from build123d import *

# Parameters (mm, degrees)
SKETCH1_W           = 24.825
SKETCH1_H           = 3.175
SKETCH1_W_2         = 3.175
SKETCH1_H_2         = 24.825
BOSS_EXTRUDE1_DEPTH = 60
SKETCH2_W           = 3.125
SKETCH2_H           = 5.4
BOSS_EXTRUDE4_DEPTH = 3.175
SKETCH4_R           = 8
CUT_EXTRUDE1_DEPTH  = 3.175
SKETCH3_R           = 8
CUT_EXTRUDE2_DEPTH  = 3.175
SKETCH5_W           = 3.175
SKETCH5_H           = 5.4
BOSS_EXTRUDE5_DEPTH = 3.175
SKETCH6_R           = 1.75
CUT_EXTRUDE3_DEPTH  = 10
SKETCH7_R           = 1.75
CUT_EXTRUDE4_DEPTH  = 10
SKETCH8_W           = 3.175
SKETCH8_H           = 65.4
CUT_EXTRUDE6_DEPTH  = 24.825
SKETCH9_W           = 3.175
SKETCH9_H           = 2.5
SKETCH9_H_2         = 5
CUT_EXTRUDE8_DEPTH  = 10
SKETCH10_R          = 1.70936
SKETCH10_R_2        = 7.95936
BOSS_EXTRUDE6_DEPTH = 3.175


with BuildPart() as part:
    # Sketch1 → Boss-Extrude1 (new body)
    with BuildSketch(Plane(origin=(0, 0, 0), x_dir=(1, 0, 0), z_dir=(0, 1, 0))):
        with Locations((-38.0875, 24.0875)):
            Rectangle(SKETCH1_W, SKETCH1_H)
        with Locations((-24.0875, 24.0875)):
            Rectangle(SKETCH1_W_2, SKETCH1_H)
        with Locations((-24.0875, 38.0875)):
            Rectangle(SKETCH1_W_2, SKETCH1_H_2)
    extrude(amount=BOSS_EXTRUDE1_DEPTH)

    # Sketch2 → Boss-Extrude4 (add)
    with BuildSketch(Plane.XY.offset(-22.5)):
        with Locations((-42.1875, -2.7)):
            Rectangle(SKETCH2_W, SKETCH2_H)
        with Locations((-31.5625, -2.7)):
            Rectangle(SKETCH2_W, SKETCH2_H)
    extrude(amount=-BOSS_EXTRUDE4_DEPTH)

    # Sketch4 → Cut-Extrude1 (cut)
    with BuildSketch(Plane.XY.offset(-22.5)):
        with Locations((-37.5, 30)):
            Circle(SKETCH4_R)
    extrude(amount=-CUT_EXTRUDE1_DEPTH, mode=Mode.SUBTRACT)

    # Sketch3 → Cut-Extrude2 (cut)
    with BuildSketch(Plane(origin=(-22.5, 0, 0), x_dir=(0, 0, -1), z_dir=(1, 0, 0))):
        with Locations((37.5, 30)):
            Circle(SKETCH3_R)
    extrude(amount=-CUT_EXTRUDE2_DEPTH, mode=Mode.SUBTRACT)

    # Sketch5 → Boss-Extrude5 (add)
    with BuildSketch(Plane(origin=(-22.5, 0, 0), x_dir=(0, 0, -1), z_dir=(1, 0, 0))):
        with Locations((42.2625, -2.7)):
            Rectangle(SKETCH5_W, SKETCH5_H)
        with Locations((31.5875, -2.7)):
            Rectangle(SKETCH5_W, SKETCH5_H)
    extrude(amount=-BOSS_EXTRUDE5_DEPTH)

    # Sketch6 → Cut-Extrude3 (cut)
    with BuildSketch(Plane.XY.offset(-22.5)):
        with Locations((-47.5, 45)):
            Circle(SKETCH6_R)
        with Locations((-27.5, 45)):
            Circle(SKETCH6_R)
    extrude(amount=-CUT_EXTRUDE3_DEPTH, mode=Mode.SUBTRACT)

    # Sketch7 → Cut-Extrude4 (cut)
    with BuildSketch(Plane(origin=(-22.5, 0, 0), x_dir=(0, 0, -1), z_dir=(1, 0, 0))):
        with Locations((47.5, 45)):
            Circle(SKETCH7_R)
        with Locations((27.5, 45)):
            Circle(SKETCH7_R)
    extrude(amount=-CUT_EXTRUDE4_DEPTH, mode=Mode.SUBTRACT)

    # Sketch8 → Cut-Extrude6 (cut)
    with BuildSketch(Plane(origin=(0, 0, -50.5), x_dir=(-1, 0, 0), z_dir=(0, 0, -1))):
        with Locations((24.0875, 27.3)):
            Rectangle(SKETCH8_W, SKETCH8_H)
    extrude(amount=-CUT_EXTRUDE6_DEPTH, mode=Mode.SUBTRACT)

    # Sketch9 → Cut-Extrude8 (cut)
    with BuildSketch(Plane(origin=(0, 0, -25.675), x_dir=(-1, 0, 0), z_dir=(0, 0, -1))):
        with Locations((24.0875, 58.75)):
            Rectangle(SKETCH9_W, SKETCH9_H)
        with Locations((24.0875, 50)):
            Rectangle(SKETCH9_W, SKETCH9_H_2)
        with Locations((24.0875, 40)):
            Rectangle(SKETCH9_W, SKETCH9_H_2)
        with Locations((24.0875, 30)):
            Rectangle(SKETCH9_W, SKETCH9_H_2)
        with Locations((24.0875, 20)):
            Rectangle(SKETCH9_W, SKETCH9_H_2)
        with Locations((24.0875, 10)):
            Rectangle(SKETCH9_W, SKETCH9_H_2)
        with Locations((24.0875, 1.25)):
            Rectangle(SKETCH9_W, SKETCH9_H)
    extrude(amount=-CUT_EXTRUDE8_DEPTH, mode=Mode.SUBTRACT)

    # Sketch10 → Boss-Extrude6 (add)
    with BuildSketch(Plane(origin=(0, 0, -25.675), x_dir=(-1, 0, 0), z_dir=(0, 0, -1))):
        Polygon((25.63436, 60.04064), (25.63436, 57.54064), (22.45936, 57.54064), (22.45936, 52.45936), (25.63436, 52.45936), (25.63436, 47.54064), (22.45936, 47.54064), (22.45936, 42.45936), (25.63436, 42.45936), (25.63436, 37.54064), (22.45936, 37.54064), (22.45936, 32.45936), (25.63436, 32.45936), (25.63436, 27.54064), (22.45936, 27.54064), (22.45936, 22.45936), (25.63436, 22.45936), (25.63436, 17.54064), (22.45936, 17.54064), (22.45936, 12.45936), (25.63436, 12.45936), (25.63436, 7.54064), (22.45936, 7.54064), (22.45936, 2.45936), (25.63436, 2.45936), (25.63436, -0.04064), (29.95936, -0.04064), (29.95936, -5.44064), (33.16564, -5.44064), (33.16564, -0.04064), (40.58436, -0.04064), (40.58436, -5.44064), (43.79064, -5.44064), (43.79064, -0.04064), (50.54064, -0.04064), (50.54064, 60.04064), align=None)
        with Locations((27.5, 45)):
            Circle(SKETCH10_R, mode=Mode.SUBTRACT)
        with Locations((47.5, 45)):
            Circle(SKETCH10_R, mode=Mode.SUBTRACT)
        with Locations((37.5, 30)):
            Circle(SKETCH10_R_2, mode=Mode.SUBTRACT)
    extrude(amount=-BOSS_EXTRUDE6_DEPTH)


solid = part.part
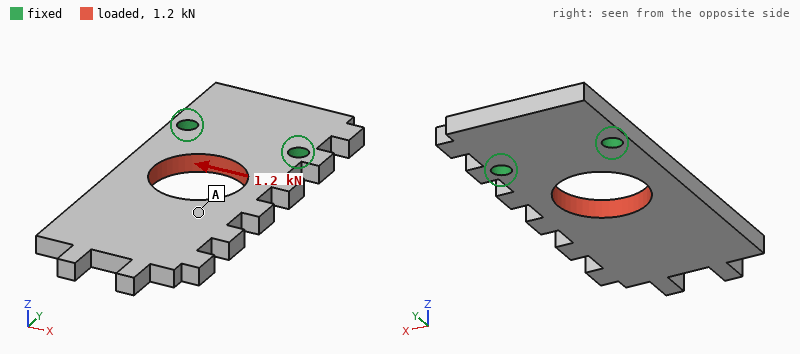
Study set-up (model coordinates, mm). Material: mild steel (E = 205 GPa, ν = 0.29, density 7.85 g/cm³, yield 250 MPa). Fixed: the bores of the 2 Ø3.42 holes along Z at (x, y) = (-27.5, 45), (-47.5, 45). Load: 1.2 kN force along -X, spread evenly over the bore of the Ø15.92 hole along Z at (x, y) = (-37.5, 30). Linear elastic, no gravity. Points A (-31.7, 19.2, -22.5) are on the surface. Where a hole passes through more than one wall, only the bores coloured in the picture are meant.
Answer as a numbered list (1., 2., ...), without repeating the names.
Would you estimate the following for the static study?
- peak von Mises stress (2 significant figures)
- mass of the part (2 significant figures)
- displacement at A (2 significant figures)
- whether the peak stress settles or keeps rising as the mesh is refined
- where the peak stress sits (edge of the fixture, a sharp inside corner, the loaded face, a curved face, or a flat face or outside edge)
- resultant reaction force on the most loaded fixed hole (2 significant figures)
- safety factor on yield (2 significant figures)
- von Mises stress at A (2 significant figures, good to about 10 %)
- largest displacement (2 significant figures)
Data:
1. 130 MPa
2. 35 g
3. 20 µm
4. settles
5. the loaded face
6. 1.0 kN
7. 1.9
8. 16 MPa
9. 25 µm
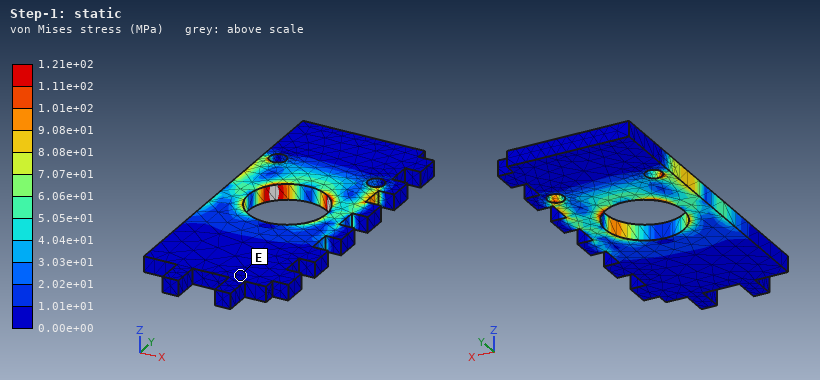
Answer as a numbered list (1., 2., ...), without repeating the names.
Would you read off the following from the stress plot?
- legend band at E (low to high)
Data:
1. 0.00e+00 to 1.01e+01 MPa
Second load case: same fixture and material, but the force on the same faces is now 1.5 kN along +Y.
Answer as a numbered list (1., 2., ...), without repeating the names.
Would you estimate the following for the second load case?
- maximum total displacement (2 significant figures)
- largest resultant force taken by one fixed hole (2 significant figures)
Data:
1. 3.7 µm
2. 760 N
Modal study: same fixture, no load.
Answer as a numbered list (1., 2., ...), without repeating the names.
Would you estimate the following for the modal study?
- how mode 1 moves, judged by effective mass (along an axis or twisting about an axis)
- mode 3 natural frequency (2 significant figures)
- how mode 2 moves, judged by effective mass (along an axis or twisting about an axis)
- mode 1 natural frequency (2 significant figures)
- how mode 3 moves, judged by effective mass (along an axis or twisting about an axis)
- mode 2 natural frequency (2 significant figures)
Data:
1. along Z
2. 5700 Hz
3. twisting about Y
4. 920 Hz
5. along X
6. 3700 Hz
